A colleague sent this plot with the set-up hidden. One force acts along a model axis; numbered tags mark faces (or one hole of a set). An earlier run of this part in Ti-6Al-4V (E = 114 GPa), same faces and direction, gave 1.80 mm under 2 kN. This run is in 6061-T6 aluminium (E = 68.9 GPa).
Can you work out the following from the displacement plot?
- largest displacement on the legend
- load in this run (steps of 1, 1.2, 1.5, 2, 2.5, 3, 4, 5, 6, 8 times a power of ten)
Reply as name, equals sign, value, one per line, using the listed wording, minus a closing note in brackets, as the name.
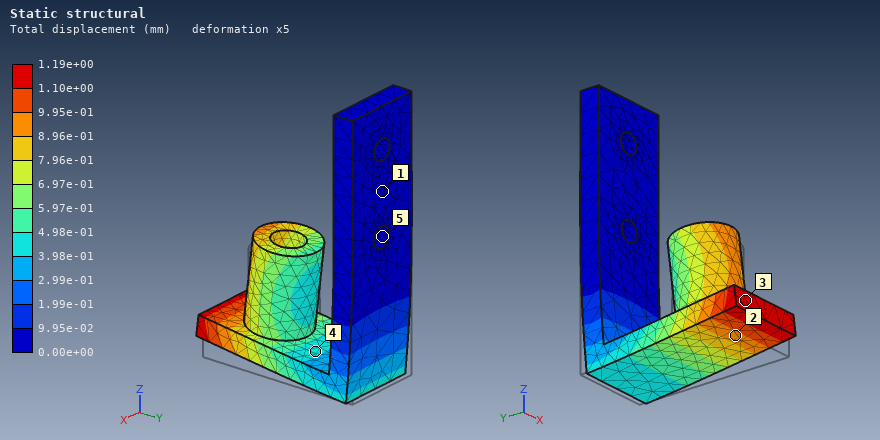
largest displacement on the legend = 1.19e+00 mm
load in this run = 800 N
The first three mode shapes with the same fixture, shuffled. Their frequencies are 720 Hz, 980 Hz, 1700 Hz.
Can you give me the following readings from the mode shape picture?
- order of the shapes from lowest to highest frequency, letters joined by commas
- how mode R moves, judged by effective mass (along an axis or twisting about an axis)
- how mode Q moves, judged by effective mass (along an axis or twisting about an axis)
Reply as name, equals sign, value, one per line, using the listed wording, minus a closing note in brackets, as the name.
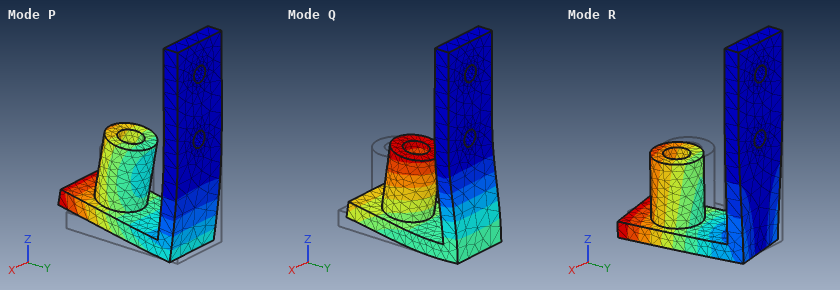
order of the shapes from lowest to highest frequency, letters joined by commas = P, R, Q
how mode R moves, judged by effective mass = along X
how mode Q moves, judged by effective mass = along Y
